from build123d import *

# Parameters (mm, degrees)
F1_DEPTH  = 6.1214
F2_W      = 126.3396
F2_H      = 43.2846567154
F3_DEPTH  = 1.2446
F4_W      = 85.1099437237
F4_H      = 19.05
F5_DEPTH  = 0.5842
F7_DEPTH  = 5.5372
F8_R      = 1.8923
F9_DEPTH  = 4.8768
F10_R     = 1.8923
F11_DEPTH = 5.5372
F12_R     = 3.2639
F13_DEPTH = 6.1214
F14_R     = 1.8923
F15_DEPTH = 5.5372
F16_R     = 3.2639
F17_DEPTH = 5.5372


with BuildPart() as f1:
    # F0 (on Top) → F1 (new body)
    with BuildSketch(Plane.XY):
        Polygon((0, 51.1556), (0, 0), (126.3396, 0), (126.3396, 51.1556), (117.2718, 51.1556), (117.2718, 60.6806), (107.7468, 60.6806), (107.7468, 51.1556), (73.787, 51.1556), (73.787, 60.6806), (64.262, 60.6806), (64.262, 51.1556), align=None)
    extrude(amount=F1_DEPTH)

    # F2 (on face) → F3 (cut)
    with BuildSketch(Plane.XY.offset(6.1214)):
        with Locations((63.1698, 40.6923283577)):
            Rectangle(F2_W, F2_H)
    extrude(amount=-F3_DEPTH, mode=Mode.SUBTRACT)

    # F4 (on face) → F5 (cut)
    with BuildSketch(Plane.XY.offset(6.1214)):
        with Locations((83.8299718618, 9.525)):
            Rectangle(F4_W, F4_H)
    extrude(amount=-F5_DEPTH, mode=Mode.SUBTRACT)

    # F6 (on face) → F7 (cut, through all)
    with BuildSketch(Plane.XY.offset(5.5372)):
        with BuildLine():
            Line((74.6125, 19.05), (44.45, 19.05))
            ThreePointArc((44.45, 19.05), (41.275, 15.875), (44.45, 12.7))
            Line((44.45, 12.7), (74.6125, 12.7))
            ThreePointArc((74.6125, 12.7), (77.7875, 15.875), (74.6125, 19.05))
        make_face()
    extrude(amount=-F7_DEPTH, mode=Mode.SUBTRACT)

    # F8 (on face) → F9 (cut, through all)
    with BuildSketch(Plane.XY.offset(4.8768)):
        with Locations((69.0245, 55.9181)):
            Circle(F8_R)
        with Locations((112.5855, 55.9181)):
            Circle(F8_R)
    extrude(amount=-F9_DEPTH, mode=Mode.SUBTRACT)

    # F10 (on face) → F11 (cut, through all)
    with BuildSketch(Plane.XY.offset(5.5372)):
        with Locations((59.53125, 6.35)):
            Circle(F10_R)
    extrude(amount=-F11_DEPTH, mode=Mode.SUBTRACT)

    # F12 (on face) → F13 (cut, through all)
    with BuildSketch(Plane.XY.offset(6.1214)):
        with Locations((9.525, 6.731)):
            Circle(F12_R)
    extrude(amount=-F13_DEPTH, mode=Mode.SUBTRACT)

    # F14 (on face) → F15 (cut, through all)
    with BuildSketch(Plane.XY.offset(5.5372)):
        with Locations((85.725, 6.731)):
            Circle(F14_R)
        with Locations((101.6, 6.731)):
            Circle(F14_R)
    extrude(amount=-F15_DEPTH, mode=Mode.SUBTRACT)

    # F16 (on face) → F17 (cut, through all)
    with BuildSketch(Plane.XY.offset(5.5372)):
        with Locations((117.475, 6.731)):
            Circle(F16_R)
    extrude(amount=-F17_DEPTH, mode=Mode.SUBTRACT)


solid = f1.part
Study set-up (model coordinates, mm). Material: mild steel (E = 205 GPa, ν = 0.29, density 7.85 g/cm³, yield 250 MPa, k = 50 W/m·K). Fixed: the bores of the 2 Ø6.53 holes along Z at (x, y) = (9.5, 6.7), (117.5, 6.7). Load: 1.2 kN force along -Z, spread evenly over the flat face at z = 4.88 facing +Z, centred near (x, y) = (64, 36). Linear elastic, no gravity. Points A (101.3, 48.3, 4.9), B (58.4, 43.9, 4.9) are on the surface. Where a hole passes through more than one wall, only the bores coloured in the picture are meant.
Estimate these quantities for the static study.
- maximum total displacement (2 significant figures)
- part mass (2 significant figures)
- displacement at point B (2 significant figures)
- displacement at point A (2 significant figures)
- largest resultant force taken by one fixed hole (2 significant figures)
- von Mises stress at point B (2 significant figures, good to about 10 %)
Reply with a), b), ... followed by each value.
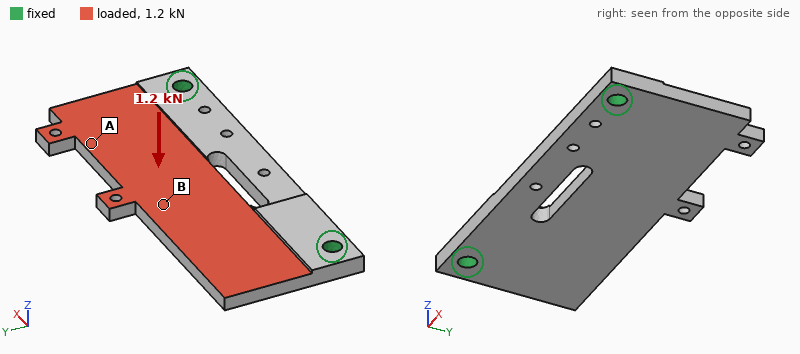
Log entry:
a) 0.20 mm
b) 260 g
c) 0.14 mm
d) 0.12 mm
e) 610 N
f) 32 MPa
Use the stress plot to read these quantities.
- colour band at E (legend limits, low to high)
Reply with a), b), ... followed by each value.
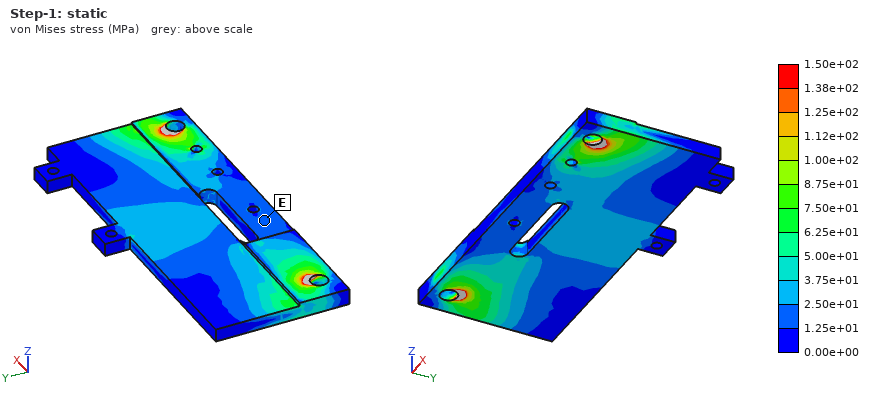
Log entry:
a) 1.25e+01 to 2.50e+01 MPa
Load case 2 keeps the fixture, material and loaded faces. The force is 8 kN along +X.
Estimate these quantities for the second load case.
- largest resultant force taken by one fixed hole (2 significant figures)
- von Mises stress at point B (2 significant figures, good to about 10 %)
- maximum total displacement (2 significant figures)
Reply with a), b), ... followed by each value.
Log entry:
a) 4.6 kN
b) 25 MPa
c) 34 µm
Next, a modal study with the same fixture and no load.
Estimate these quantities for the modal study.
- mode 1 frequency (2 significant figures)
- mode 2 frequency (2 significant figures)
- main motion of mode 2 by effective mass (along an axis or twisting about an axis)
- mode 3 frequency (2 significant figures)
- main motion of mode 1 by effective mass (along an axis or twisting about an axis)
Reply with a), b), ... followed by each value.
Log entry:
a) 1300 Hz
b) 2500 Hz
c) twisting about Y
d) 2900 Hz
e) along Z
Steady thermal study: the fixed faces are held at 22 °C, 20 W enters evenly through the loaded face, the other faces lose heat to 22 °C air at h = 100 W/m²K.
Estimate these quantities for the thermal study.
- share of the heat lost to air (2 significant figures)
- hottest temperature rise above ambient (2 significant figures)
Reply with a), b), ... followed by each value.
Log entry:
a) 58 %
b) 18 K
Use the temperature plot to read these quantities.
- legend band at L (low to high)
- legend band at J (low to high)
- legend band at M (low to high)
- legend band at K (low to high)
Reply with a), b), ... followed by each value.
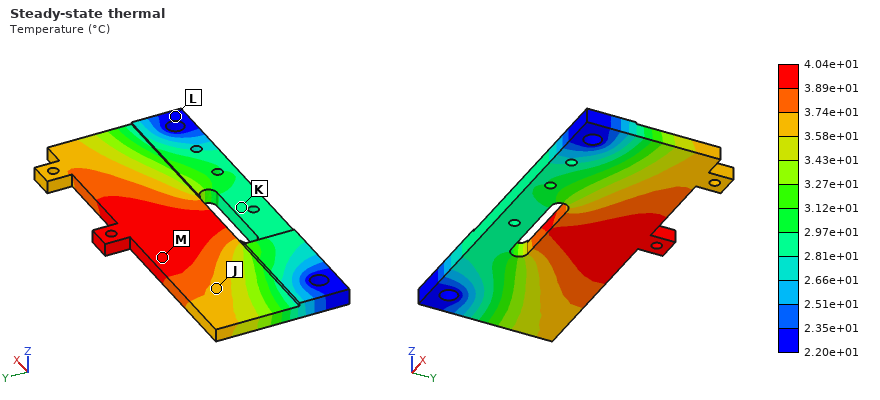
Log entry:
a) 2.20e+01 to 2.35e+01 °C
b) 3.58e+01 to 3.74e+01 °C
c) 3.89e+01 to 4.04e+01 °C
d) 2.81e+01 to 2.97e+01 °C
